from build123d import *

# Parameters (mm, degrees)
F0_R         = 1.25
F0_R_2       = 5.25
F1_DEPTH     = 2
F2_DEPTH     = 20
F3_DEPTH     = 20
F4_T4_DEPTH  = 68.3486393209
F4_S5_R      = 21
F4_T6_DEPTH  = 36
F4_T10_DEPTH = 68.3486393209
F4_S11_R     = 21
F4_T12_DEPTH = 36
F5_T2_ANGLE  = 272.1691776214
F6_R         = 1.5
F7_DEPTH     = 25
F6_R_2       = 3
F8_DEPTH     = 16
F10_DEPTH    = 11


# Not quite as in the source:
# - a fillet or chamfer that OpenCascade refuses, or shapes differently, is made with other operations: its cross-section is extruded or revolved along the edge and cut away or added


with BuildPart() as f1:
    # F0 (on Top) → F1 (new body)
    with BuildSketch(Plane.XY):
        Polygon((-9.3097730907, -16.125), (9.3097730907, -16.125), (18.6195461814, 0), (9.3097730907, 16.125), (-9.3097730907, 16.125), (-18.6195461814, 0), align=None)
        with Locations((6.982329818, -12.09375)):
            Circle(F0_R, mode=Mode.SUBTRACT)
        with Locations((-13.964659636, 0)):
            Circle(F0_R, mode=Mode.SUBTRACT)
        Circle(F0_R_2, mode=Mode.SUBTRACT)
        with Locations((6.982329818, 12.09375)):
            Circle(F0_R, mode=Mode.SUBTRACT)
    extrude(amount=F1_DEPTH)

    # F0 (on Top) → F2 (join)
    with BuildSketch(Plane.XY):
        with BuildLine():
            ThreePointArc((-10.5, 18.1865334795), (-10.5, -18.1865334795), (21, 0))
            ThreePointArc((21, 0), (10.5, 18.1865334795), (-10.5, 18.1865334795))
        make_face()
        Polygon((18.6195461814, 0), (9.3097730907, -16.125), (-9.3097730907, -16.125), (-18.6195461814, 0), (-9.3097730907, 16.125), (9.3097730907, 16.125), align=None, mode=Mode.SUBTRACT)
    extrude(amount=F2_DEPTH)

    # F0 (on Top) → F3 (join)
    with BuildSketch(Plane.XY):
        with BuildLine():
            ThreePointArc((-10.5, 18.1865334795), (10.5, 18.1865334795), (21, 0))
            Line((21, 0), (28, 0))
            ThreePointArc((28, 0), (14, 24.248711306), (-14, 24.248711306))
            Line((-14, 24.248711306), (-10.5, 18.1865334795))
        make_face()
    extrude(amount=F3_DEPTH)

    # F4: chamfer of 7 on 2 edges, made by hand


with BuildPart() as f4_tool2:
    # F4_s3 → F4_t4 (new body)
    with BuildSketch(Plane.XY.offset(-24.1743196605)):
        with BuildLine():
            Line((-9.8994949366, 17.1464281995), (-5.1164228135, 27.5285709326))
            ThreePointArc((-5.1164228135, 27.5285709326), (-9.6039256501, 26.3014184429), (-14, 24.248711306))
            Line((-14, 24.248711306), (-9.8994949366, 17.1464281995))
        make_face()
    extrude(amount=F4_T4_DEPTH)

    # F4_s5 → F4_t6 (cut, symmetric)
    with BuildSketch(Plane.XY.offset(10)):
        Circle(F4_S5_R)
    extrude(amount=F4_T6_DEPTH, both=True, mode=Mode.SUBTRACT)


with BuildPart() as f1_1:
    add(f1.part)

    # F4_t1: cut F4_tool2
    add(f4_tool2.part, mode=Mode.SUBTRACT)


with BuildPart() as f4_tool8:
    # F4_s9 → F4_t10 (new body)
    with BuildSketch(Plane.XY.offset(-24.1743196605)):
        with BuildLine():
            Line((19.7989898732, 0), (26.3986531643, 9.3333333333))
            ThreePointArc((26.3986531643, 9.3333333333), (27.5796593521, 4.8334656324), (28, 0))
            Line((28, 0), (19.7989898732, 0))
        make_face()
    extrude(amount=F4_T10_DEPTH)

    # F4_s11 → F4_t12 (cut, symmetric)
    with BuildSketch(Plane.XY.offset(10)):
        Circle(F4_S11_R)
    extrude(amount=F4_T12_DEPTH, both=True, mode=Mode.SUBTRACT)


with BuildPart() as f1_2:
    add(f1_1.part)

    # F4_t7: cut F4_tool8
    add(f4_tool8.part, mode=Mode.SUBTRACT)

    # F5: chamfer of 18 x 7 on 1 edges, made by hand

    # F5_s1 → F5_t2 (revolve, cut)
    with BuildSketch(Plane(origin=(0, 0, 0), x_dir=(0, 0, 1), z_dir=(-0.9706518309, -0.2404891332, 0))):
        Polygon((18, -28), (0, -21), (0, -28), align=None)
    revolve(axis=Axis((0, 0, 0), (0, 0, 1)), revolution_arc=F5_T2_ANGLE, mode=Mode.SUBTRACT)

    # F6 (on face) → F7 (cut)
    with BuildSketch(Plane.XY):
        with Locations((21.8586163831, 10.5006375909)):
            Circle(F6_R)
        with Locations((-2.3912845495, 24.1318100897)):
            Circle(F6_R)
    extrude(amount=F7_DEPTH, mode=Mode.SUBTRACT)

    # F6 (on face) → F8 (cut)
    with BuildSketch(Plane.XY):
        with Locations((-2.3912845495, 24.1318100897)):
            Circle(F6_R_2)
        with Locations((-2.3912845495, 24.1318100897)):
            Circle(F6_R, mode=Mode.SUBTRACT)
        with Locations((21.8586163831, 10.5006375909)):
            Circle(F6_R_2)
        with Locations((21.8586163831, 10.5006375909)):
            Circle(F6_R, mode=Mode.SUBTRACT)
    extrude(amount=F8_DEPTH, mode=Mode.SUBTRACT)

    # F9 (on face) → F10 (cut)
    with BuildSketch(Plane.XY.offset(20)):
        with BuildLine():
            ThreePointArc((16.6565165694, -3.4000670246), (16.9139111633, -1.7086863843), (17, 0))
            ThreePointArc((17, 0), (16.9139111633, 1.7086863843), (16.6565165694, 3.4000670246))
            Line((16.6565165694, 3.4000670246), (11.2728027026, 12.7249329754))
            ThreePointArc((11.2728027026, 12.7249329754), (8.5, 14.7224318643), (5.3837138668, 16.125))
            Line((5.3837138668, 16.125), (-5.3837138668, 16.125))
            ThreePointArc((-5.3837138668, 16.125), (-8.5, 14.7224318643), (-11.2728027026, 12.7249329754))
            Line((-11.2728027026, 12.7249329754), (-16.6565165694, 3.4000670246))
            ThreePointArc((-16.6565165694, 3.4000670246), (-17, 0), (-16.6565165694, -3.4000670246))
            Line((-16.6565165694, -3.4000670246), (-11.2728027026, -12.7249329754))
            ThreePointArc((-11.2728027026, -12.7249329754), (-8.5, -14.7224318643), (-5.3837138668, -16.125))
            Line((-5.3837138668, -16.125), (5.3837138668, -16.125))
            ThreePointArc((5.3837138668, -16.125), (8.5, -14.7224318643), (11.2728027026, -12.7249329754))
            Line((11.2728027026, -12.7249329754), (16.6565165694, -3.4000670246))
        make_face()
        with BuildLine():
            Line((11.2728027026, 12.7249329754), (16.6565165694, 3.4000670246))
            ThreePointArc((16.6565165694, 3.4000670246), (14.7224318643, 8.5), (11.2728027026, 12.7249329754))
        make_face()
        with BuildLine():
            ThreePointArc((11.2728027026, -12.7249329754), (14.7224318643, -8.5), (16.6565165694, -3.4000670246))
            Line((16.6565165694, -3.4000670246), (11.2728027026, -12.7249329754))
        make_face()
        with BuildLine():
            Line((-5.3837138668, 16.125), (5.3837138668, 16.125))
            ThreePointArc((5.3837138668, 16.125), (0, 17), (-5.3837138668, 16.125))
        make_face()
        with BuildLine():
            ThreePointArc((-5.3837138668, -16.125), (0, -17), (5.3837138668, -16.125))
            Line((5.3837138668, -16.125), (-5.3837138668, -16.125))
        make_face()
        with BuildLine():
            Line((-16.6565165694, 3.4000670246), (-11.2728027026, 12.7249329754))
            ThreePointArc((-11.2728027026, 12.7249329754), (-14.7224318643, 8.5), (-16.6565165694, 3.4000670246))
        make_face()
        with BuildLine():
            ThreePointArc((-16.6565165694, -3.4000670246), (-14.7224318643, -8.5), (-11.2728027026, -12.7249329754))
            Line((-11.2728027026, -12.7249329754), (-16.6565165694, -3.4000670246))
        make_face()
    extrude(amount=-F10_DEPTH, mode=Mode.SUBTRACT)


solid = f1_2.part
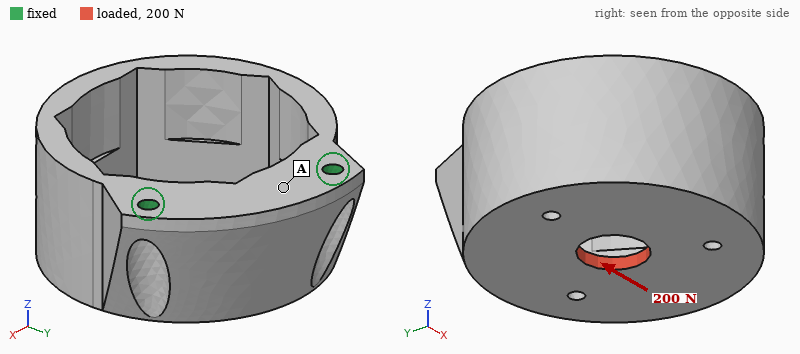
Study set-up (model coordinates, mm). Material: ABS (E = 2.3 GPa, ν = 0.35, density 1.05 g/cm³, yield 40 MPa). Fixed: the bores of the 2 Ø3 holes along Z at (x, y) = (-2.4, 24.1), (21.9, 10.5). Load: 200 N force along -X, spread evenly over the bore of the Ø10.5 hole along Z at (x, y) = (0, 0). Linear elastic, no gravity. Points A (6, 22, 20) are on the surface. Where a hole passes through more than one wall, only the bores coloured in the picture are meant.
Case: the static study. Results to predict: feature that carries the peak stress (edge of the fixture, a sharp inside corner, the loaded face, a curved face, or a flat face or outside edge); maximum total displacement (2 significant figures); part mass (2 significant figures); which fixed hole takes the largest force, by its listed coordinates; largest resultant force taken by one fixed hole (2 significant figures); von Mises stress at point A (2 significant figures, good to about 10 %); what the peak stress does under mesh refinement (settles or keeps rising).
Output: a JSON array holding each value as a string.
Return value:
["edge of the fixture", "0.71 mm", "14 g", "(21.9, 10.5)", "210 N", "4.1 MPa", "keeps rising"]
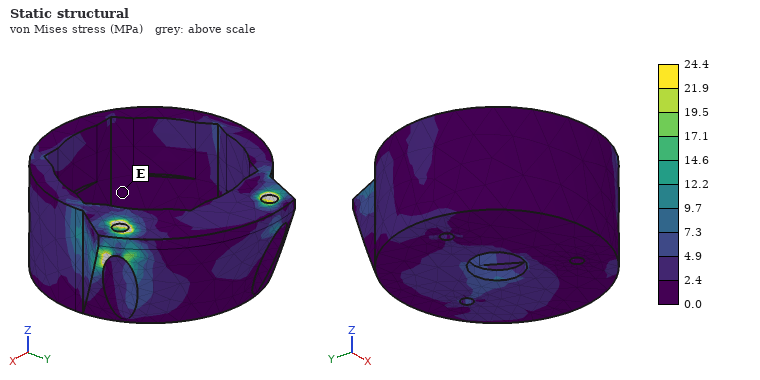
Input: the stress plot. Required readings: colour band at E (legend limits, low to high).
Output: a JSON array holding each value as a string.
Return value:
["0.0 to 2.4 MPa"]
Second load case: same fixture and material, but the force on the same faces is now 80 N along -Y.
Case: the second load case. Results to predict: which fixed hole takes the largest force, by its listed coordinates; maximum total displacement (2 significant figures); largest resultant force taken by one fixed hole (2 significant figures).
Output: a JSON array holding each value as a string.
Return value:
["(-2.4, 24.1)", "0.43 mm", "66 N"]
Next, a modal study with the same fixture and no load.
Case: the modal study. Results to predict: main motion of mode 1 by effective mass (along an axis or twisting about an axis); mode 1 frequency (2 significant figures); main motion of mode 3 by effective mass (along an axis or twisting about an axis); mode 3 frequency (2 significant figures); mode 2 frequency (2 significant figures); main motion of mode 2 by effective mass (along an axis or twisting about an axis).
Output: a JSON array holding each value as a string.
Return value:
["along Z", "620 Hz", "along Y", "2400 Hz", "960 Hz", "along X"]
